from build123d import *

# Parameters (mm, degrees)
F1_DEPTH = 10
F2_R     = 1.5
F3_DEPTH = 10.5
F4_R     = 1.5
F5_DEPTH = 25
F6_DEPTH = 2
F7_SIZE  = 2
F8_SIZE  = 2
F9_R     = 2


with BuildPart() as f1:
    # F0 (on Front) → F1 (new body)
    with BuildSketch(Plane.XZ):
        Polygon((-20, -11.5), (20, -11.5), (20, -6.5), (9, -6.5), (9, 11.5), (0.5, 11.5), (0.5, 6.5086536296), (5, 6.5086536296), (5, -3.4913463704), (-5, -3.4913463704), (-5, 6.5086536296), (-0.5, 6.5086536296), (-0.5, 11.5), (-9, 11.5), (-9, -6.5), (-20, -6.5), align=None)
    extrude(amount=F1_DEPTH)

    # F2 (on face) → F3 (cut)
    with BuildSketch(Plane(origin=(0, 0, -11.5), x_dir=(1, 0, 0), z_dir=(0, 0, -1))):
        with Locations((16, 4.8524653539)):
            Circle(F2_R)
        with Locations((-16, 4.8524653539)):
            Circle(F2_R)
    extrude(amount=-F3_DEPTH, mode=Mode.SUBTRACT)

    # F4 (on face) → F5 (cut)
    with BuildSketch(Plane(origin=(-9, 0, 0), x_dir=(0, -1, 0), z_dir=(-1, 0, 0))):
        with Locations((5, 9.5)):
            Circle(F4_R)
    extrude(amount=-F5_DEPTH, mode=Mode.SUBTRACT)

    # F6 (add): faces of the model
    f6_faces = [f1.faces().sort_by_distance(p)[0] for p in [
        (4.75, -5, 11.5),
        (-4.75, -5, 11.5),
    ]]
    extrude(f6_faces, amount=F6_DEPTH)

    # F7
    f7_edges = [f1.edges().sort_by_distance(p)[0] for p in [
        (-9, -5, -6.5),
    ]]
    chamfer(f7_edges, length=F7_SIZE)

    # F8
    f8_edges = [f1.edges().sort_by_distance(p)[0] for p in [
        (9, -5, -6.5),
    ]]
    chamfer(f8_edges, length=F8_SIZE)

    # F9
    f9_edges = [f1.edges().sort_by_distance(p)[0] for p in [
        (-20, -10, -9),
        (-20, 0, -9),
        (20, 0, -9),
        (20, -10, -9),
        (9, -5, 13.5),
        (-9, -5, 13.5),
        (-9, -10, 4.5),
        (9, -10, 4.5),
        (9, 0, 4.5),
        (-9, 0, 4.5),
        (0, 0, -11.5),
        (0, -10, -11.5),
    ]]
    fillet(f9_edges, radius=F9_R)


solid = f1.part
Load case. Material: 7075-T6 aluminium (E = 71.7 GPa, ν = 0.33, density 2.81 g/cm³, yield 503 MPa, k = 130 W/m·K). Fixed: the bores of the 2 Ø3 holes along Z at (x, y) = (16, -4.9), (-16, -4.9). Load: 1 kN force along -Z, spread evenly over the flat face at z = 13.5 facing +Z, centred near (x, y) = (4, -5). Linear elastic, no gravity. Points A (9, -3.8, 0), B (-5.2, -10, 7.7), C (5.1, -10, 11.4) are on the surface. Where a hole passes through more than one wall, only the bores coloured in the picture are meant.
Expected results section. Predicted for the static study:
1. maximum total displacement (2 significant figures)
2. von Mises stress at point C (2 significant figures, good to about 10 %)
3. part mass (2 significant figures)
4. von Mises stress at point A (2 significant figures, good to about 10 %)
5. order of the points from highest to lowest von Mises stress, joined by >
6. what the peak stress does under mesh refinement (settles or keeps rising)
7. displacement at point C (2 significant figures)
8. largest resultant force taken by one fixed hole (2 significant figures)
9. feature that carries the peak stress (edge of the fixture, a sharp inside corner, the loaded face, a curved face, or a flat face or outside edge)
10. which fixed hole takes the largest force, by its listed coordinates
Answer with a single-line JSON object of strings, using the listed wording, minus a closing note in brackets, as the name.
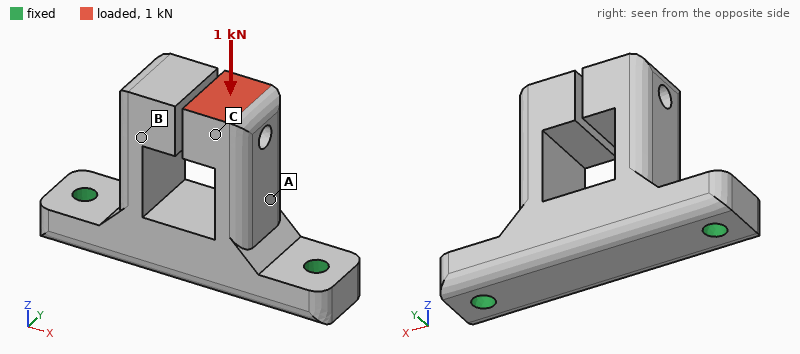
{"maximum total displacement": "0.19 mm", "von Mises stress at point C": "28 MPa", "part mass": "12 g", "von Mises stress at point A": "100 MPa", "order of the points from highest to lowest von Mises stress, joined by >": "A > C > B", "what the peak stress does under mesh refinement": "keeps rising", "displacement at point C": "0.13 mm", "largest resultant force taken by one fixed hole": "740 N", "feature that carries the peak stress": "edge of the fixture", "which fixed hole takes the largest force, by its listed coordinates": "(16, -4.9)"}
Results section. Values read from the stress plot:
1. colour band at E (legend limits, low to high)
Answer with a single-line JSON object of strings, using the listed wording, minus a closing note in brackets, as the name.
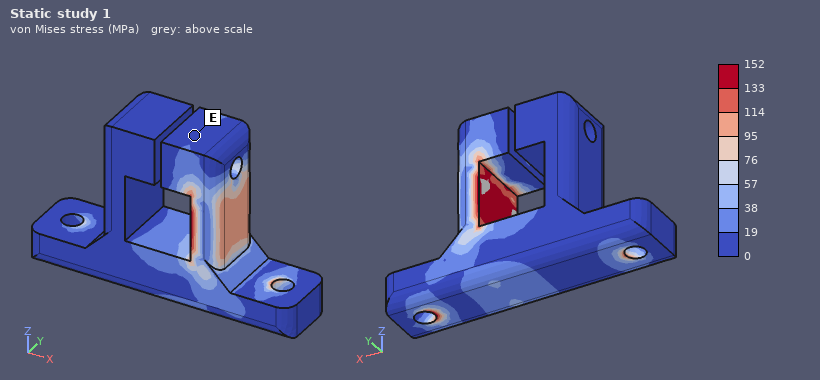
{"colour band at E": "0 to 19 MPa"}
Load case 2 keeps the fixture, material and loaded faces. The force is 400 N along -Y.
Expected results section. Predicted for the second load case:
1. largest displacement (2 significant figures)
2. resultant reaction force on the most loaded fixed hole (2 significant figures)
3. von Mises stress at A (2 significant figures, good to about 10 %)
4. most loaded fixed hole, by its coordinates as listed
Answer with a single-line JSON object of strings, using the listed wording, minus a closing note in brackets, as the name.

{"largest displacement": "0.18 mm", "resultant reaction force on the most loaded fixed hole": "260 N", "von Mises stress at A": "32 MPa", "most loaded fixed hole, by its coordinates as listed": "(16, -4.9)"}
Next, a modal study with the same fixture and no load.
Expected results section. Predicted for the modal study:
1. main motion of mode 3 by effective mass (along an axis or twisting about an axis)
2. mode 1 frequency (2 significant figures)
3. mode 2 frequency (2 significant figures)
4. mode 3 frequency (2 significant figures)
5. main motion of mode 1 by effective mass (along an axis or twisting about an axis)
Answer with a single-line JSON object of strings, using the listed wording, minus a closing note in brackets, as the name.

{"main motion of mode 3 by effective mass": "along X", "mode 1 frequency": "5700 Hz", "mode 2 frequency": "6000 Hz", "mode 3 frequency": "6300 Hz", "main motion of mode 1 by effective mass": "along Y"}
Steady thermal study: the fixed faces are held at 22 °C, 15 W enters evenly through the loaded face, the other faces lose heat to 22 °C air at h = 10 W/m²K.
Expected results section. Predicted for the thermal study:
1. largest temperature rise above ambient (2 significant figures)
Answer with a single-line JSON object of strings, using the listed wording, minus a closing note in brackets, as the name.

{"largest temperature rise above ambient": "66 K"}
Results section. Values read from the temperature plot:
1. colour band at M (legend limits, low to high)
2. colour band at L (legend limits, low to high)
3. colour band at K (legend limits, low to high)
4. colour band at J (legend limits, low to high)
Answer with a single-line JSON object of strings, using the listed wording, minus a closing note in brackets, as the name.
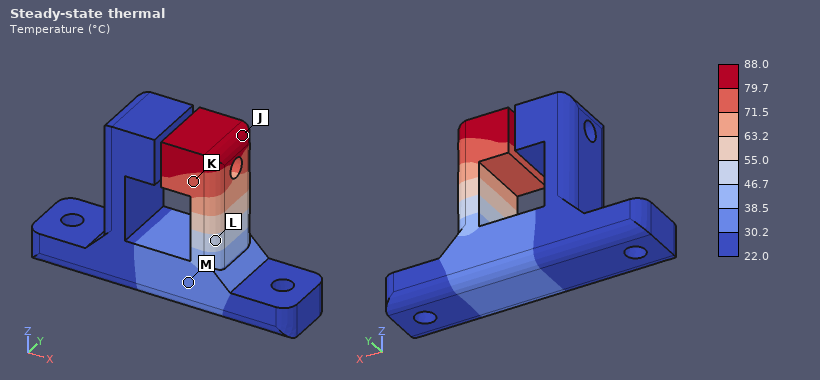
{"colour band at M": "30.2 to 38.5 °C", "colour band at L": "46.7 to 55.0 °C", "colour band at K": "71.5 to 79.7 °C", "colour band at J": "79.7 to 88.0 °C"}
